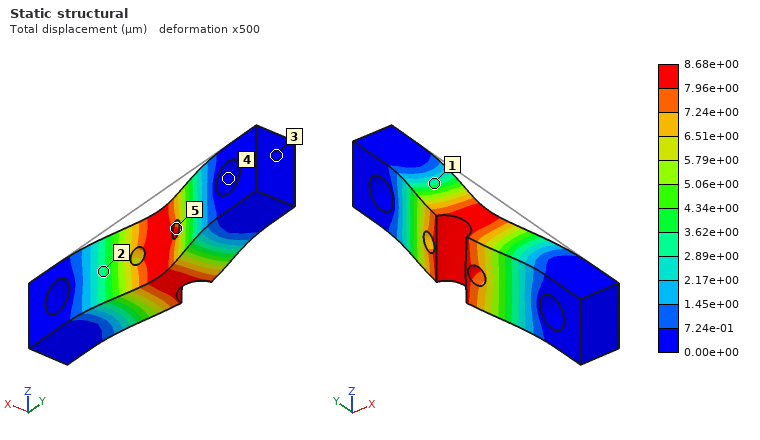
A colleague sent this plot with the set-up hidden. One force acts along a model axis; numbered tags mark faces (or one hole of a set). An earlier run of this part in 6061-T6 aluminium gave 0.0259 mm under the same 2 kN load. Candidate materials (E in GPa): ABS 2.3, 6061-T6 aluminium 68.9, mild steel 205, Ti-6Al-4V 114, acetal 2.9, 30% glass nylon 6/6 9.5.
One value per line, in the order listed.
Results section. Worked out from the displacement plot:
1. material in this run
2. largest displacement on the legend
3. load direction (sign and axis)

mild steel
8.68e+00 µm
-X
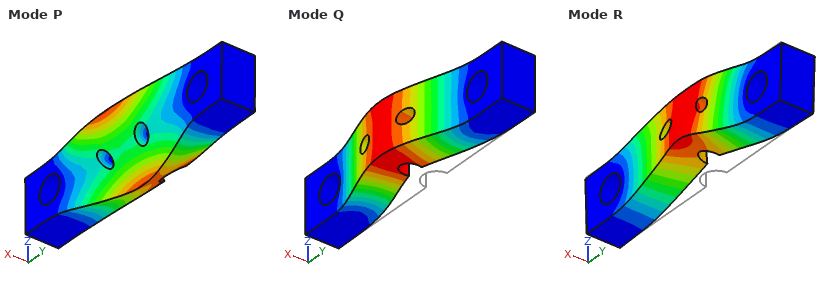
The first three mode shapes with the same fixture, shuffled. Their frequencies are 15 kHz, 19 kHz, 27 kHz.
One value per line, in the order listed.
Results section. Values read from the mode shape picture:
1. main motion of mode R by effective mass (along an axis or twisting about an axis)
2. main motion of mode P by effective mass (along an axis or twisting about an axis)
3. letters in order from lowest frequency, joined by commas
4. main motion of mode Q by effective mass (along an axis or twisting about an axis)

along Z
twisting about Y
Q, R, P
along X
